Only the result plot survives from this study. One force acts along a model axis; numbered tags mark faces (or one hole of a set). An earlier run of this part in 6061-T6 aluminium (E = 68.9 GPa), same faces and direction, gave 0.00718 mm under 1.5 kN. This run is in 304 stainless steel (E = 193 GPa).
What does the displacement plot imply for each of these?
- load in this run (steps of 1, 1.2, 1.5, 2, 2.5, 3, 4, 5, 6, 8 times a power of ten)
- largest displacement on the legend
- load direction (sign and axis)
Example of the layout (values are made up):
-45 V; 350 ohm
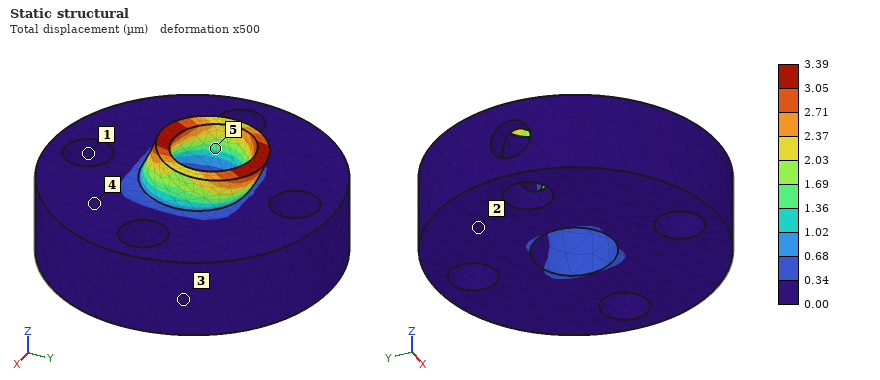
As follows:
2 kN; 3.39 µm; +Y
